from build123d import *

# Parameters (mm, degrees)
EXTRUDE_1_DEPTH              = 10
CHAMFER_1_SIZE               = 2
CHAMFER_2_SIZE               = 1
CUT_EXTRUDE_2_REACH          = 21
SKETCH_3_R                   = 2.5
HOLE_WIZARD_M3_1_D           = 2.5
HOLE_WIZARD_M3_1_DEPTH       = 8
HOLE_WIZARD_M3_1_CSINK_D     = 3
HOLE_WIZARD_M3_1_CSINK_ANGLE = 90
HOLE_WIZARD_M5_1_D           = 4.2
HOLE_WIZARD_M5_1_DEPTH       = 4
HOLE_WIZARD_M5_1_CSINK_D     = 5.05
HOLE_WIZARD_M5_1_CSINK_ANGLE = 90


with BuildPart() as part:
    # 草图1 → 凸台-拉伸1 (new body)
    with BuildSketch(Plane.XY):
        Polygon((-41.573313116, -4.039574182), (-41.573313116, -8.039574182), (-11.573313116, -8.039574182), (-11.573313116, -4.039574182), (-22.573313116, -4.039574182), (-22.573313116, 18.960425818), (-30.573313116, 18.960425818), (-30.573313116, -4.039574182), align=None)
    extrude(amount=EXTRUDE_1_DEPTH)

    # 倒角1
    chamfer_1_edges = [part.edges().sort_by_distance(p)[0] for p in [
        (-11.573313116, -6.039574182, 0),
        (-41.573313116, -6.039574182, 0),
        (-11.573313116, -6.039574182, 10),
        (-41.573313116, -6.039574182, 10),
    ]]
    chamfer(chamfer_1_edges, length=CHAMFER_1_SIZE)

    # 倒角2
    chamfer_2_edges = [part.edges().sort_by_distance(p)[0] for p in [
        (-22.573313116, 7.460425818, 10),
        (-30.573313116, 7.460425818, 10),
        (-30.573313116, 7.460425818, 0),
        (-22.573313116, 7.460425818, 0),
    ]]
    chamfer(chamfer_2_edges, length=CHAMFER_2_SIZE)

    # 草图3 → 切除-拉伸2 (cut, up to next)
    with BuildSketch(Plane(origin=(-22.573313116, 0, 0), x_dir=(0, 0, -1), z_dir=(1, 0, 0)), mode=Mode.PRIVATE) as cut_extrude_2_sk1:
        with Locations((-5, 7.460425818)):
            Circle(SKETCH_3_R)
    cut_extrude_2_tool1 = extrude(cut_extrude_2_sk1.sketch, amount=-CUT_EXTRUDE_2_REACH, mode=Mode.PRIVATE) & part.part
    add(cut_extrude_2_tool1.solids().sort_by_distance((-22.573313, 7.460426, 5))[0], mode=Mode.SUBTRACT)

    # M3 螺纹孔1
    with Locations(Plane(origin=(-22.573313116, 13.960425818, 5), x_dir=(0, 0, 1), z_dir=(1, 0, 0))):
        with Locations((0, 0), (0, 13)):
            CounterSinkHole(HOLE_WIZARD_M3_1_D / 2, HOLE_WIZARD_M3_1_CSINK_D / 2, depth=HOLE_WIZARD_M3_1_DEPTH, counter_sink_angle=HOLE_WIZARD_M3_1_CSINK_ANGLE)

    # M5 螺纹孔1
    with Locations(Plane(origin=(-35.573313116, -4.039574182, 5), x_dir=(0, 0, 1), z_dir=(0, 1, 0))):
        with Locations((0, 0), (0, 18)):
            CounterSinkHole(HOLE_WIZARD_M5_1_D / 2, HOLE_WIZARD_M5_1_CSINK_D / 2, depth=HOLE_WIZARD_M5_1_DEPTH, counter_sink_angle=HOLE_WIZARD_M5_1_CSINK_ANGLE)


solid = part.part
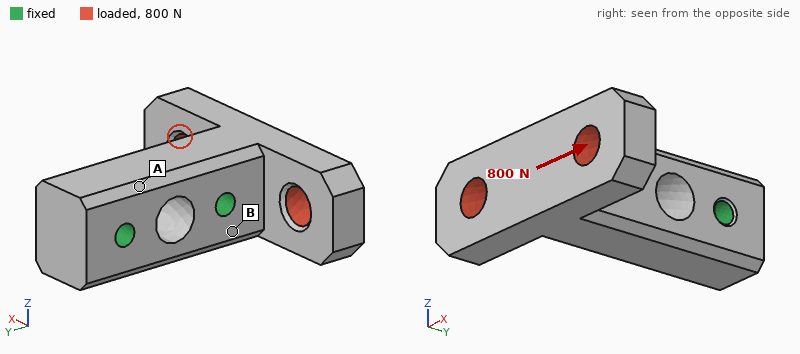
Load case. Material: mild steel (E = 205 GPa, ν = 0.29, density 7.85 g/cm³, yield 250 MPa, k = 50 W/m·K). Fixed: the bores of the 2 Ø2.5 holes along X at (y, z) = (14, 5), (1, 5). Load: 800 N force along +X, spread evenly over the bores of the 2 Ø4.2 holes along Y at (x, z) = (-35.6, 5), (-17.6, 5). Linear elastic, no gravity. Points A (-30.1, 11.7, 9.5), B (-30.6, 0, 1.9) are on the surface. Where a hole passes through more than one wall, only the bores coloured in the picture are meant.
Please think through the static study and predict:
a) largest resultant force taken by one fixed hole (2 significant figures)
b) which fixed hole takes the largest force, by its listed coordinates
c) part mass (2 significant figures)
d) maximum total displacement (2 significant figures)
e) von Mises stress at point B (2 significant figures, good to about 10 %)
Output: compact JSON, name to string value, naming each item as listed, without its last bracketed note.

{"largest resultant force taken by one fixed hole": "860 N", "which fixed hole takes the largest force, by its listed coordinates": "(1, 5)", "part mass": "21 g", "maximum total displacement": "6.8 µm", "von Mises stress at point B": "30 MPa"}
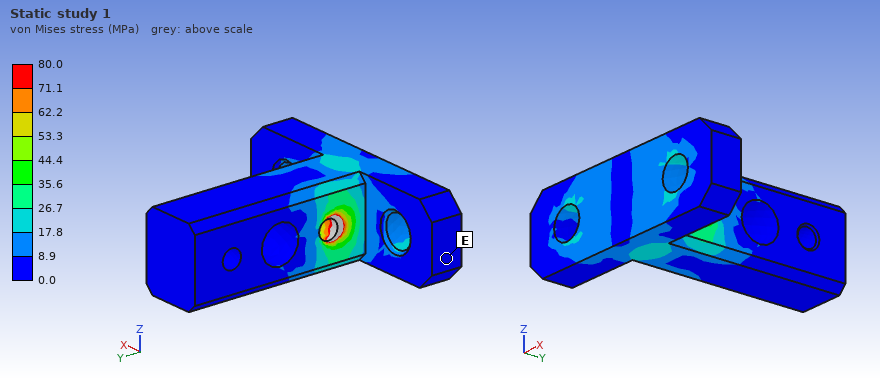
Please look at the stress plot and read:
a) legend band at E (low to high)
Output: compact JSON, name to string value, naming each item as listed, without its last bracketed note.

{"legend band at E": "0.0 to 8.9 MPa"}
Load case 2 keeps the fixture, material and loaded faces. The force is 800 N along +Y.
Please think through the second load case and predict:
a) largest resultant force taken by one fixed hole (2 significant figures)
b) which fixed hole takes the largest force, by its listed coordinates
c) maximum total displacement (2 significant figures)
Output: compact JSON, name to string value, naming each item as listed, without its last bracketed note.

{"largest resultant force taken by one fixed hole": "730 N", "which fixed hole takes the largest force, by its listed coordinates": "(1, 5)", "maximum total displacement": "12 µm"}
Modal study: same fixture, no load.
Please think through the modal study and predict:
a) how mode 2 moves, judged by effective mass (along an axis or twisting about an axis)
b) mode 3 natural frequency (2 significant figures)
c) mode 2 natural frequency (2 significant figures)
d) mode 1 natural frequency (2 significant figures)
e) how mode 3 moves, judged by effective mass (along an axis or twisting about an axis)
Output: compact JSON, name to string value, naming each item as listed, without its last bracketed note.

{"how mode 2 moves, judged by effective mass": "twisting about Y", "mode 3 natural frequency": "19 kHz", "mode 2 natural frequency": "18 kHz", "mode 1 natural frequency": "15 kHz", "how mode 3 moves, judged by effective mass": "along Y"}
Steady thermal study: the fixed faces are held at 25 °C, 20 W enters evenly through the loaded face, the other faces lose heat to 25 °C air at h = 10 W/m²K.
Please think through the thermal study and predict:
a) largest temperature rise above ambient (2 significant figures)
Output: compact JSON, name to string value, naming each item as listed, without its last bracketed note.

{"largest temperature rise above ambient": "75 K"}
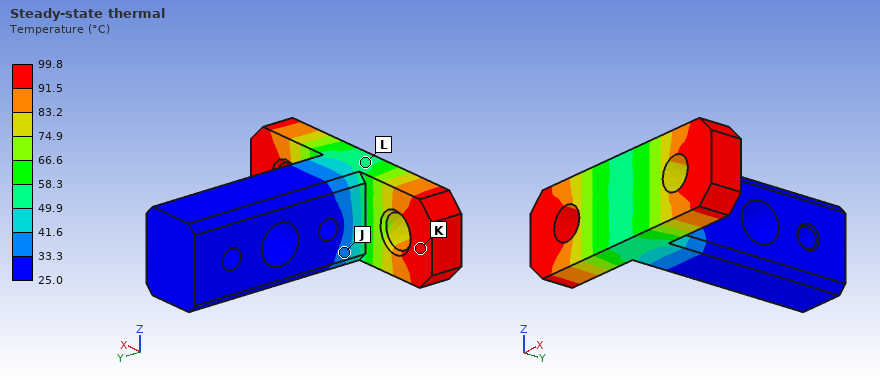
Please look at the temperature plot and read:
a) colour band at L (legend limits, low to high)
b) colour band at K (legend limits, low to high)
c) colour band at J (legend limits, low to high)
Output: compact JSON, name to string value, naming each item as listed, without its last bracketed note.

{"colour band at L": "49.9 to 58.3 °C", "colour band at K": "91.5 to 99.8 °C", "colour band at J": "33.3 to 41.6 °C"}
